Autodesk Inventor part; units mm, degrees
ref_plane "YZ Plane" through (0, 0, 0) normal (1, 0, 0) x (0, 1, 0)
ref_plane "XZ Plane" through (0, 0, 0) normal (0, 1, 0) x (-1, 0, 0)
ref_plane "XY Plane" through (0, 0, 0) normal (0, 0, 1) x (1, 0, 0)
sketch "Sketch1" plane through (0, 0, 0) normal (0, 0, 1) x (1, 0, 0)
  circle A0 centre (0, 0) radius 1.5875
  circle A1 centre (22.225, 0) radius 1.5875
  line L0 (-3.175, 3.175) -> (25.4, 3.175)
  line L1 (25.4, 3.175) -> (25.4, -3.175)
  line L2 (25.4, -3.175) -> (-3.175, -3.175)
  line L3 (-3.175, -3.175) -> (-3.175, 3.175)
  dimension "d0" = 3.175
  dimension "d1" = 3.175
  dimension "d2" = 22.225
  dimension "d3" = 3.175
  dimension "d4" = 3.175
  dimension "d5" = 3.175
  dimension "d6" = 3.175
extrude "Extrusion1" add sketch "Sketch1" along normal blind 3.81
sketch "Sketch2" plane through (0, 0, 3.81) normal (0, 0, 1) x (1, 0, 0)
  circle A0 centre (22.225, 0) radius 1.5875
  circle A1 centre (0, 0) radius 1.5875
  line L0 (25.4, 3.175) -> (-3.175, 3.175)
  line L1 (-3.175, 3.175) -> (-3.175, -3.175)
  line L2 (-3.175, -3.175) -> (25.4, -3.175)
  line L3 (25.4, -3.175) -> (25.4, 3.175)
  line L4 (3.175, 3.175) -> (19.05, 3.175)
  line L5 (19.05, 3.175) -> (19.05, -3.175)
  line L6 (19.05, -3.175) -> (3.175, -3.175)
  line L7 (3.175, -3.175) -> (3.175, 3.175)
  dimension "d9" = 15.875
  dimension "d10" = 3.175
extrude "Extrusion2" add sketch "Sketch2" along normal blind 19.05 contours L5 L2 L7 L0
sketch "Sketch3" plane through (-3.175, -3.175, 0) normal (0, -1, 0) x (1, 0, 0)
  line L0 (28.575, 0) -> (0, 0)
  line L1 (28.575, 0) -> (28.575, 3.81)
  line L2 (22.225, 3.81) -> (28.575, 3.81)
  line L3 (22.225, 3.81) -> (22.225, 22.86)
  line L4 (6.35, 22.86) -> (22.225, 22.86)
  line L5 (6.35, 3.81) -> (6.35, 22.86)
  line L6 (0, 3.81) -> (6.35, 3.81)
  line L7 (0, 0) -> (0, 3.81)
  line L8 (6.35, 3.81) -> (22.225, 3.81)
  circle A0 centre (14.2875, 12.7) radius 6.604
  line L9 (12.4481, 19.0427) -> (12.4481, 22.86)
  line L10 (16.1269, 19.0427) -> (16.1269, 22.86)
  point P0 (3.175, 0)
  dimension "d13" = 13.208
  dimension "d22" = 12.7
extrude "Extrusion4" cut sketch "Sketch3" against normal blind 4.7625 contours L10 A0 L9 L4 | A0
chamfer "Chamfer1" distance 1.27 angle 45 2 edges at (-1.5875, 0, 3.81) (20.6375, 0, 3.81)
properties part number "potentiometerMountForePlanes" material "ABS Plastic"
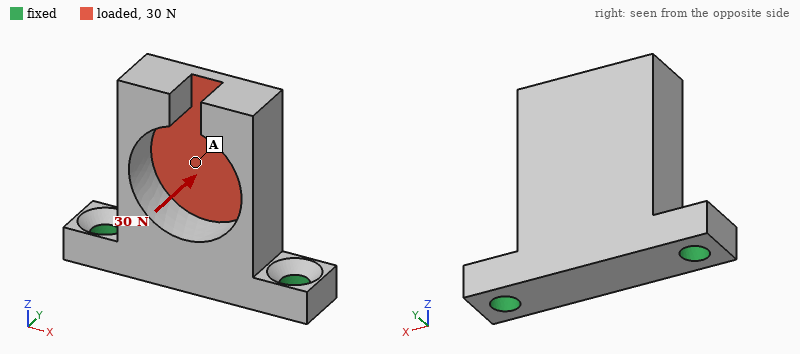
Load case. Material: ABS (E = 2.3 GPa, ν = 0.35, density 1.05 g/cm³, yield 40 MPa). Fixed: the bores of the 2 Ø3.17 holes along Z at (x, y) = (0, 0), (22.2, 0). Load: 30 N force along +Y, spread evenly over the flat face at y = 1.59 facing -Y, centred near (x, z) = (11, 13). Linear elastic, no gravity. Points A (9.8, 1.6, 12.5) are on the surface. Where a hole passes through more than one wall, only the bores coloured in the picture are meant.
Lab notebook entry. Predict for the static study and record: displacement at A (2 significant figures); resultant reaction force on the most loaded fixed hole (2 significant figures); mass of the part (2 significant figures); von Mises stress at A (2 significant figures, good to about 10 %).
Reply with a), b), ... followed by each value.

a) 0.19 mm
b) 15 N
c) 1.9 g
d) 3.0 MPa
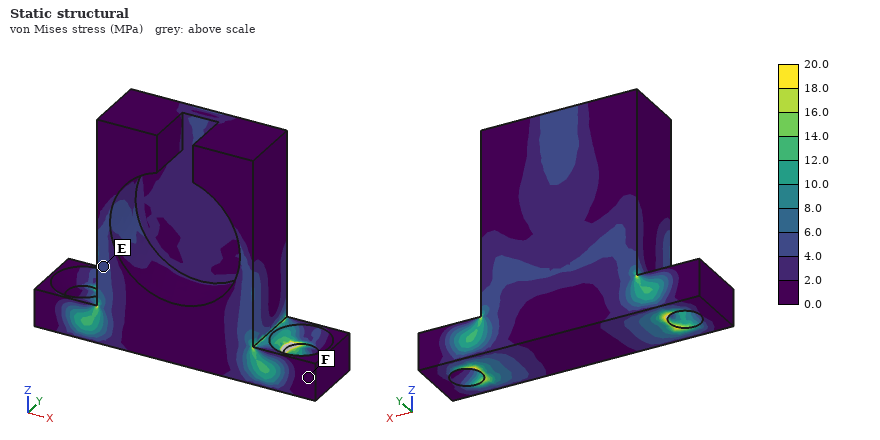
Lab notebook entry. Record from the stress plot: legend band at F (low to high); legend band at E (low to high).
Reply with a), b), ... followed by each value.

a) 0.0 to 2.0 MPa
b) 4.0 to 6.0 MPa
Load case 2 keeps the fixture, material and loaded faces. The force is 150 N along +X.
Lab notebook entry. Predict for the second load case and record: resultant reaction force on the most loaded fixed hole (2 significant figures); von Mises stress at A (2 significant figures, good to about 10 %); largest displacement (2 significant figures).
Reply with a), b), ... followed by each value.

a) 120 N
b) 8.1 MPa
c) 0.25 mm
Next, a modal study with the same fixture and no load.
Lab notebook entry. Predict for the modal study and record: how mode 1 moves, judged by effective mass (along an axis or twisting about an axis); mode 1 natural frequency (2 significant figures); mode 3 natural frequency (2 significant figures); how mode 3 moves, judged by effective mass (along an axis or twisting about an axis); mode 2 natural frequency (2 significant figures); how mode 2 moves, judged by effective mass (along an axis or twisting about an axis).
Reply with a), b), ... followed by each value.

a) along Y
b) 1500 Hz
c) 5500 Hz
d) along X
e) 3200 Hz
f) along X
